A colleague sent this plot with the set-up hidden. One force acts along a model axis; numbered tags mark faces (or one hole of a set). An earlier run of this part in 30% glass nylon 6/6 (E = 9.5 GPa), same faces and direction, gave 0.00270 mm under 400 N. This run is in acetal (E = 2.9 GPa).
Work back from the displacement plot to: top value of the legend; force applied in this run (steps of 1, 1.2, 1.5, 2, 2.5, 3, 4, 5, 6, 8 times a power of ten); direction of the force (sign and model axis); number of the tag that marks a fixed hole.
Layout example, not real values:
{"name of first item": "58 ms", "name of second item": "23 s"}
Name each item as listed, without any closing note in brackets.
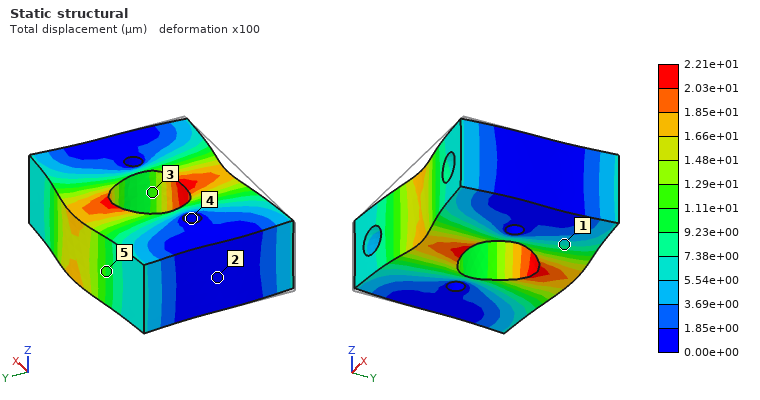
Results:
{"top value of the legend": "2.21e+01 µm", "force applied in this run": "1 kN", "direction of the force": "+Y", "number of the tag that marks a fixed hole": "4"}
